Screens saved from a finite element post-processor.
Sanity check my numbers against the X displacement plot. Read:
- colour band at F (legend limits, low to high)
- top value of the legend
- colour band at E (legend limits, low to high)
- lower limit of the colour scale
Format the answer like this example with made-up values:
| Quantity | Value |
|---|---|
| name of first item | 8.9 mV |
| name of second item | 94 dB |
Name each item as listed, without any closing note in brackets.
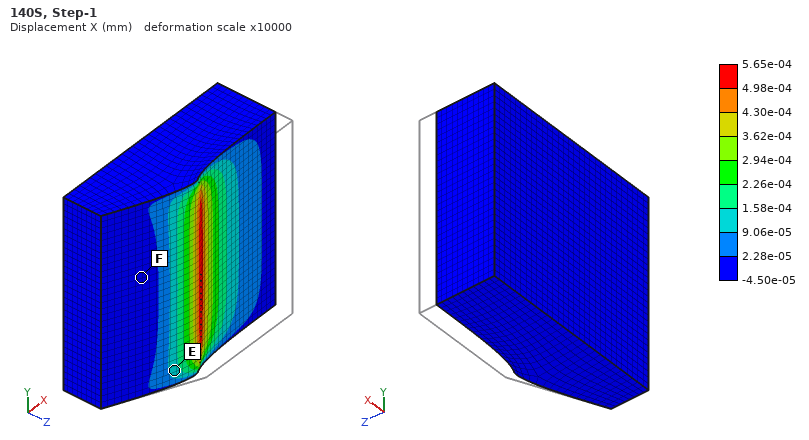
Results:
| Quantity | Value |
|---|---|
| colour band at F | -4.50e-05 to 2.28e-05 mm |
| top value of the legend | 5.65e-04 mm |
| colour band at E | 9.06e-05 to 1.58e-04 mm |
| lower limit of the colour scale | -4.50e-05 mm |
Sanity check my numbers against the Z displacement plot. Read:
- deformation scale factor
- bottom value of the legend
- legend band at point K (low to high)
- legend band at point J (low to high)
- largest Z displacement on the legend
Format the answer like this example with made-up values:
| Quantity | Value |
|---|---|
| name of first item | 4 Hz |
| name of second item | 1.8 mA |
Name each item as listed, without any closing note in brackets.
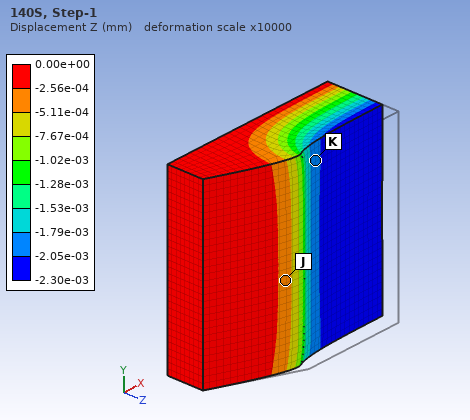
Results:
| Quantity | Value |
|---|---|
| deformation scale factor | 10000 |
| bottom value of the legend | -2.30e-03 mm |
| legend band at point K | -2.05e-03 to -1.79e-03 mm |
| legend band at point J | -5.11e-04 to -2.56e-04 mm |
| largest Z displacement on the legend | 0.00e+00 mm |
